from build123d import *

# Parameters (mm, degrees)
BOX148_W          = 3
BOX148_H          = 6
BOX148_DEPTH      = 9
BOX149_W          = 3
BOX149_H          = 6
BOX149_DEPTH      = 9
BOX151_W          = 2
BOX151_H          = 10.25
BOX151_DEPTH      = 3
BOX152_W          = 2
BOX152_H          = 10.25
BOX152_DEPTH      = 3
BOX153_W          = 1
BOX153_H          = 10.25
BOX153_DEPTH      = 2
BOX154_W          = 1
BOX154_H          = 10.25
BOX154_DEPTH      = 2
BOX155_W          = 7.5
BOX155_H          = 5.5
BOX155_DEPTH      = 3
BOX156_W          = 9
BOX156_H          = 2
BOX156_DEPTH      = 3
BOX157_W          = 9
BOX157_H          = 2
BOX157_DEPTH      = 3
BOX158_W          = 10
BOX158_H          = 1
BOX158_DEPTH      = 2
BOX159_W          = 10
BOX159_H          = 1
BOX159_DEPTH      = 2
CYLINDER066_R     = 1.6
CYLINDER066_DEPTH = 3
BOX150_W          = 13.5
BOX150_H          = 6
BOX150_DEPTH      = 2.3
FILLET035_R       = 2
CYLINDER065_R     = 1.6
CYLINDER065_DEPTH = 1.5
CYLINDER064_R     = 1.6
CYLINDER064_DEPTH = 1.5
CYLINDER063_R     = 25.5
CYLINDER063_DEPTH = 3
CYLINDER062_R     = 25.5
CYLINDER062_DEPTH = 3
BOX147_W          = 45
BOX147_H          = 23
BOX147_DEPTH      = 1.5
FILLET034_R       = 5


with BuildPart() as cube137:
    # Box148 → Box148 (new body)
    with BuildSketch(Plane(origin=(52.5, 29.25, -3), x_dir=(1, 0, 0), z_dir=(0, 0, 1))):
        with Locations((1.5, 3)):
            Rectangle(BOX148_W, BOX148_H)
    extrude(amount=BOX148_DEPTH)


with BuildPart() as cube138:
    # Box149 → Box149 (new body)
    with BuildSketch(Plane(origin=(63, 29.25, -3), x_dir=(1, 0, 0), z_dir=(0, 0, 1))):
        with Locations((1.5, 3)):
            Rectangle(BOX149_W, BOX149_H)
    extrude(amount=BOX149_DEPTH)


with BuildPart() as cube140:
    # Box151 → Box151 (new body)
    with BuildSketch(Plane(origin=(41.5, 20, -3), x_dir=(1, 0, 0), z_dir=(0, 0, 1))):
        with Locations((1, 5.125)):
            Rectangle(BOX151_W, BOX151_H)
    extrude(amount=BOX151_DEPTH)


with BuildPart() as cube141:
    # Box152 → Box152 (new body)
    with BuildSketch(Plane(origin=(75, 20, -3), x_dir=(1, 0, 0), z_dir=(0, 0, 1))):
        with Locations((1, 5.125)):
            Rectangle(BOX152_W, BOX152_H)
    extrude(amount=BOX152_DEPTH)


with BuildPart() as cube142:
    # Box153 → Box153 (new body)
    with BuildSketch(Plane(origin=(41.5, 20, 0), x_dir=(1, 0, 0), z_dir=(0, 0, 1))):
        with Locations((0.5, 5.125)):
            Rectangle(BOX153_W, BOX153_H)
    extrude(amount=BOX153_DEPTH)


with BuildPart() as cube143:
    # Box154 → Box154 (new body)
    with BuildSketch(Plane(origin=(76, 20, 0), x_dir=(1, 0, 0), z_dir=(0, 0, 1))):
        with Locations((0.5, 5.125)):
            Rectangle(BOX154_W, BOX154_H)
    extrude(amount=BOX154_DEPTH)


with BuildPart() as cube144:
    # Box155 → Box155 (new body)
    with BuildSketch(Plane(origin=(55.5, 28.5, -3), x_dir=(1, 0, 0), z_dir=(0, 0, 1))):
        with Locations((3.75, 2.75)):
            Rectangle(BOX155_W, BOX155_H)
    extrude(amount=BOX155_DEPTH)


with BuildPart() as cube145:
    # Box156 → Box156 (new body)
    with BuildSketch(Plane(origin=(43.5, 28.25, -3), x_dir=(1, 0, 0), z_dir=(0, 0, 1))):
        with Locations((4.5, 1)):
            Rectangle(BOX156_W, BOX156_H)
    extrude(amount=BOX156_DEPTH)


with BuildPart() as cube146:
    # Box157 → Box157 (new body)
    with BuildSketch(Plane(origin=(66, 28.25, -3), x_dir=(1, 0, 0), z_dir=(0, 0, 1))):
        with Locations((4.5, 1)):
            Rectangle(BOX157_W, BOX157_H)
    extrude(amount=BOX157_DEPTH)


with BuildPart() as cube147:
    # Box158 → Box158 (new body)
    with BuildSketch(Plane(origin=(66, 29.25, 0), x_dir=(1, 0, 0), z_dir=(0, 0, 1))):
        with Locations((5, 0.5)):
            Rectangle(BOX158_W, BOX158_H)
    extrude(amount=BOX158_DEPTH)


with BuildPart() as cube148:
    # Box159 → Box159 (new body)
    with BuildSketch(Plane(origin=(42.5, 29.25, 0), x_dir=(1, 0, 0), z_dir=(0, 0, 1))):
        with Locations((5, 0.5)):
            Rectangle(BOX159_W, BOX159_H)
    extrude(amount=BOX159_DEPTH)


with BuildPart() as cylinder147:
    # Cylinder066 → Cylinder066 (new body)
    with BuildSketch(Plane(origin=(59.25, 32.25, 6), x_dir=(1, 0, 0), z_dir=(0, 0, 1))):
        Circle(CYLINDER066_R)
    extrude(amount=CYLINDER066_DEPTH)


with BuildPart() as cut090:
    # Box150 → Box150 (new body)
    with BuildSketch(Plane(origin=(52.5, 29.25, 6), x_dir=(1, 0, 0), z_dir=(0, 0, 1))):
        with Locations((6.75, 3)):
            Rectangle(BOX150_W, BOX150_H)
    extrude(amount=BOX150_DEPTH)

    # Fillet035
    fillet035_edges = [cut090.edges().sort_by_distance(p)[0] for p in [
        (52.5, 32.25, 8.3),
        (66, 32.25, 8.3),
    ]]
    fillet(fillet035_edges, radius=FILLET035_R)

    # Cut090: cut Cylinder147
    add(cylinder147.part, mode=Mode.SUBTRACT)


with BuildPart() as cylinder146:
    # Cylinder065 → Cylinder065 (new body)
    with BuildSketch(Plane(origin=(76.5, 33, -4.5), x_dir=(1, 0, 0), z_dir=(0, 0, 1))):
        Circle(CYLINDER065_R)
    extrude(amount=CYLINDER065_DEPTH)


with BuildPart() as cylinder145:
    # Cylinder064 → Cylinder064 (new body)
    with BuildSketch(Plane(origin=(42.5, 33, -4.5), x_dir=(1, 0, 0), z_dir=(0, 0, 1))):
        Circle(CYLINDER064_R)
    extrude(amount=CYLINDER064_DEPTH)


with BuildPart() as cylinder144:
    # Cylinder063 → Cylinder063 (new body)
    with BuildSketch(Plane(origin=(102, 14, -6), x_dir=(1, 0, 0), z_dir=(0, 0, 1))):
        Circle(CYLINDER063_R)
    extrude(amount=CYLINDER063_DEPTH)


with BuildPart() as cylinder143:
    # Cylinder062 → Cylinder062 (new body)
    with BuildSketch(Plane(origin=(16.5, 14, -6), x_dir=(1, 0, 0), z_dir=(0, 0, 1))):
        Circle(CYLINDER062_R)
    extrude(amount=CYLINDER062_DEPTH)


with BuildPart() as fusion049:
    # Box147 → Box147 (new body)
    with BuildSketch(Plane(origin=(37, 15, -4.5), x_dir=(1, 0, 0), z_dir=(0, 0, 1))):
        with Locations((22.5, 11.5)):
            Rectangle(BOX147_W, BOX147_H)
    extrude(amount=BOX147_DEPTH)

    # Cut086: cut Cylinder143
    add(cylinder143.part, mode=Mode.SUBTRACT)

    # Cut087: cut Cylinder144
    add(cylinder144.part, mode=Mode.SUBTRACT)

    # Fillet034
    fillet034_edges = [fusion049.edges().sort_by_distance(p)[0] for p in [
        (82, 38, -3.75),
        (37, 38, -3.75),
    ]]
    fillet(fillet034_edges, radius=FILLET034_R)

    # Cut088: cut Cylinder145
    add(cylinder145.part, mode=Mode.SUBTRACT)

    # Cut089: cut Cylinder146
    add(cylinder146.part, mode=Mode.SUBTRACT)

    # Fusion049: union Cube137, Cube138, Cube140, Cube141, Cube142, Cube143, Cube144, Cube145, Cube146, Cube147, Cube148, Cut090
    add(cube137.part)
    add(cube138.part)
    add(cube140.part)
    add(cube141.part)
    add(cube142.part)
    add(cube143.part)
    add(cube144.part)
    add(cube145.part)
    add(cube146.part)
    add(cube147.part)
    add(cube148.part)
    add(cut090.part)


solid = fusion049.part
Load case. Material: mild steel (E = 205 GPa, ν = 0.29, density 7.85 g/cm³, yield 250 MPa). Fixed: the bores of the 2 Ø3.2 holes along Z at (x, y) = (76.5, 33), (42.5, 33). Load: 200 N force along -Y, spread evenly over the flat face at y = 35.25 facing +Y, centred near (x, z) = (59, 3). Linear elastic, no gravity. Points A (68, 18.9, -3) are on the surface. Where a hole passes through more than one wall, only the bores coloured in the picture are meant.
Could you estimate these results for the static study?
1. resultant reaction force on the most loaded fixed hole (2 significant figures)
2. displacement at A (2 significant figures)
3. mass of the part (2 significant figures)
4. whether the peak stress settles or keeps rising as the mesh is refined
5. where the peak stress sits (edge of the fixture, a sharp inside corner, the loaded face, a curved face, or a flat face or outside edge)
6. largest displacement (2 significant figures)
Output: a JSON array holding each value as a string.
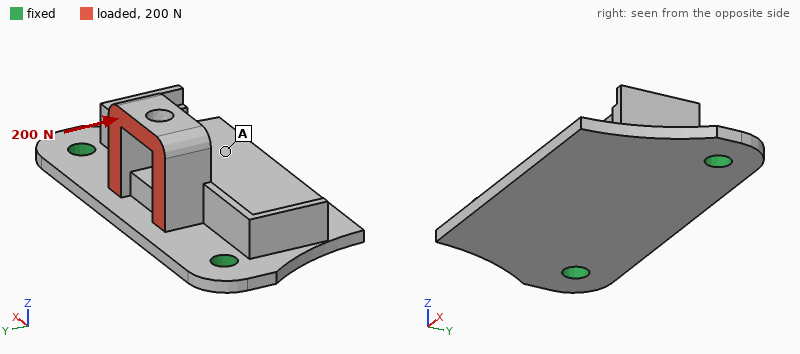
["100 N", "30 µm", "18 g", "keeps rising", "edge of the fixture", "44 µm"]
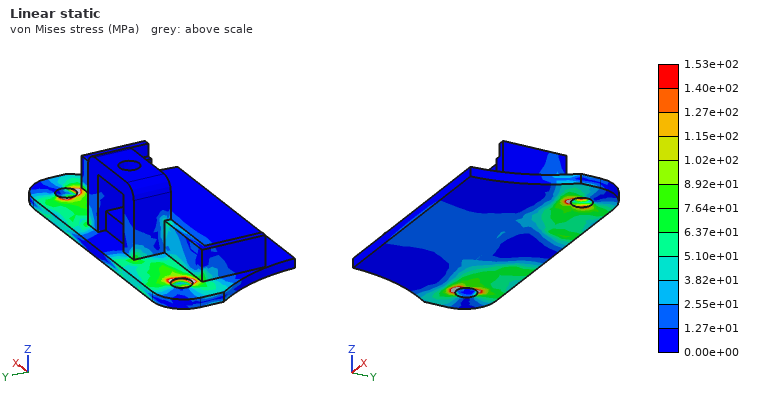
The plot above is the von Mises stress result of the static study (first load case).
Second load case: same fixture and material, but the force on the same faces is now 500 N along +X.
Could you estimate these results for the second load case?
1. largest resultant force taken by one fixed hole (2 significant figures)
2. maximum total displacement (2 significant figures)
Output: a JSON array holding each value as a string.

["280 N", "12 µm"]
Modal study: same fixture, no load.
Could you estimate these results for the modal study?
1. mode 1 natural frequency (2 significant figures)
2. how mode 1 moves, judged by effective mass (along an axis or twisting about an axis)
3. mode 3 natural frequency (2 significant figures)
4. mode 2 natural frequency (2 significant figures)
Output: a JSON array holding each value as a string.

["3600 Hz", "along Z", "7900 Hz", "7800 Hz"]
